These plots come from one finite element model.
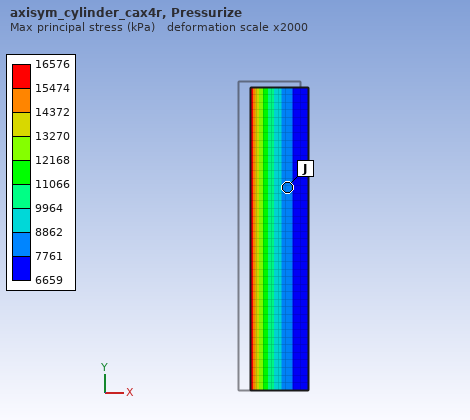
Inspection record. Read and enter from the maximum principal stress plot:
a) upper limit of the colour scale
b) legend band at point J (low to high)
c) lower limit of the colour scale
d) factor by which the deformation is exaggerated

16576 kPa
7761 to 8862 kPa
6659 kPa
2000
